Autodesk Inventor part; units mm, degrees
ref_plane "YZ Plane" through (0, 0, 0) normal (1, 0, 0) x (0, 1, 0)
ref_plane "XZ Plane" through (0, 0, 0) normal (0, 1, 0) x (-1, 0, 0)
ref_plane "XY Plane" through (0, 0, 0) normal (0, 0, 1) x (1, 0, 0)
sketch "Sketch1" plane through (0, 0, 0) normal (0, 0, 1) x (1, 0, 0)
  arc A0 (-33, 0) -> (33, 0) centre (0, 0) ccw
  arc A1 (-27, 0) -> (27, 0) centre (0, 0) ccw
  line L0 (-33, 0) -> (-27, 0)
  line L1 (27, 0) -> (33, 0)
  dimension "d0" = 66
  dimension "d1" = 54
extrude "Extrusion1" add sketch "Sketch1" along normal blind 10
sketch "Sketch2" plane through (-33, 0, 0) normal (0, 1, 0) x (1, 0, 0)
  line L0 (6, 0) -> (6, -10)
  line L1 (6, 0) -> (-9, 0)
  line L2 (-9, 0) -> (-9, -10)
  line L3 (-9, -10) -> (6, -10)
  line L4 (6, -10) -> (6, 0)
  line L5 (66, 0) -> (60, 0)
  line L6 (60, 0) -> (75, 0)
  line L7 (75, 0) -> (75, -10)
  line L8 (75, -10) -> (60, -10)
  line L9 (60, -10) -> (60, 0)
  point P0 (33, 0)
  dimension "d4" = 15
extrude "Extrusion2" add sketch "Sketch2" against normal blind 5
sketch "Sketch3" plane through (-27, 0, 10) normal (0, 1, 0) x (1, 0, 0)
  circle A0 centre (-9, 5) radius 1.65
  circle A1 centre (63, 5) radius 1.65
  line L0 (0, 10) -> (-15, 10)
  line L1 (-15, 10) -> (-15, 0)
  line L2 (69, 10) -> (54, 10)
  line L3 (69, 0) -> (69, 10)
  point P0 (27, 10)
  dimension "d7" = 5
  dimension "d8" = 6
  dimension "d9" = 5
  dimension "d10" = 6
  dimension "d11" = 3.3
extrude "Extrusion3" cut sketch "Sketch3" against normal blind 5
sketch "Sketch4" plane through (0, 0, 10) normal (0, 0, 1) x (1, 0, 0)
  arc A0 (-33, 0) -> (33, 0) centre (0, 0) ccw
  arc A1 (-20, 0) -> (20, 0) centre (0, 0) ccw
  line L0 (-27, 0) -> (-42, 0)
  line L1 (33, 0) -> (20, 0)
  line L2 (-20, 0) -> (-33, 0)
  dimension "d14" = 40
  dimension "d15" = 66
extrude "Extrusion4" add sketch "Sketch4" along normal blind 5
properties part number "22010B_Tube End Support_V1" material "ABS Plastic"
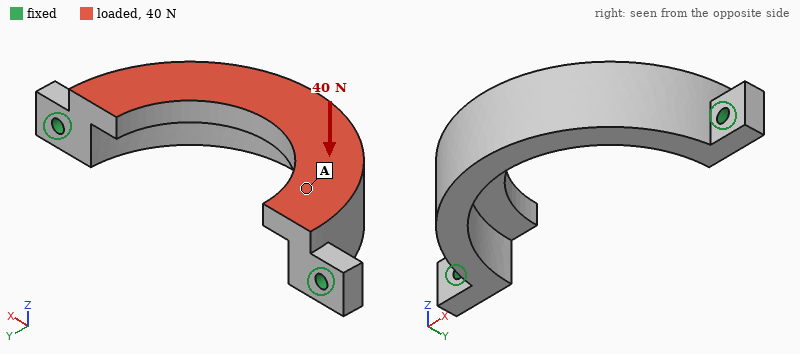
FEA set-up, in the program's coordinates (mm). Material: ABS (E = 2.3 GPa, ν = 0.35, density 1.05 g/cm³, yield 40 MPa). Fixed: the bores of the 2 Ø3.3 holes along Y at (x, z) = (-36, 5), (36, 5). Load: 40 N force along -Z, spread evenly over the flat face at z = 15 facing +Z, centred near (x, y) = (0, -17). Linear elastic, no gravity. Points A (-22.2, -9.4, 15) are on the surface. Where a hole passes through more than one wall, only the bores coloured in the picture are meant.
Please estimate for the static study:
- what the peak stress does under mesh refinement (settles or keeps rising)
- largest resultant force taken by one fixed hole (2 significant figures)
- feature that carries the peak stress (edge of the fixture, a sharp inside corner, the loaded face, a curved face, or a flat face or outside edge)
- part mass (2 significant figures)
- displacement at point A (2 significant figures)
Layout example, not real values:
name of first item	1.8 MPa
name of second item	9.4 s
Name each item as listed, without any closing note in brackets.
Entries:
what the peak stress does under mesh refinement	keeps rising
largest resultant force taken by one fixed hole	20 N
feature that carries the peak stress	edge of the fixture
part mass	12 g
displacement at point A	0.075 mm
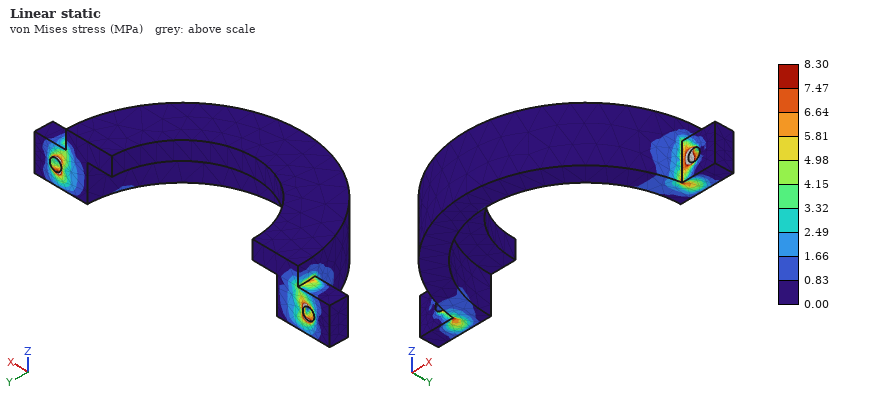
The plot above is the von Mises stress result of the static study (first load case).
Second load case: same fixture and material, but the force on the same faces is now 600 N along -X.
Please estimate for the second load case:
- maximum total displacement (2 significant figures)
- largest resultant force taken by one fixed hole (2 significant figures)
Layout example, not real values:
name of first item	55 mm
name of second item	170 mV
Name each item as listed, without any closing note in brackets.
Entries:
maximum total displacement	0.31 mm
largest resultant force taken by one fixed hole	330 N
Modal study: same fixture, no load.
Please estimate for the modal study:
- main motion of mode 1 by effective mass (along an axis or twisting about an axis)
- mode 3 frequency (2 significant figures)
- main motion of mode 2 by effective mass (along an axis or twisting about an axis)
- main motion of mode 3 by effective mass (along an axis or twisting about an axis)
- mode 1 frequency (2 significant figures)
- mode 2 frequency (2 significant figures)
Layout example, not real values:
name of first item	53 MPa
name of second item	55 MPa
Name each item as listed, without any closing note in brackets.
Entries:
main motion of mode 1 by effective mass	along Z
mode 3 frequency	3000 Hz
main motion of mode 2 by effective mass	along X
main motion of mode 3 by effective mass	along X
mode 1 frequency	760 Hz
mode 2 frequency	2200 Hz
